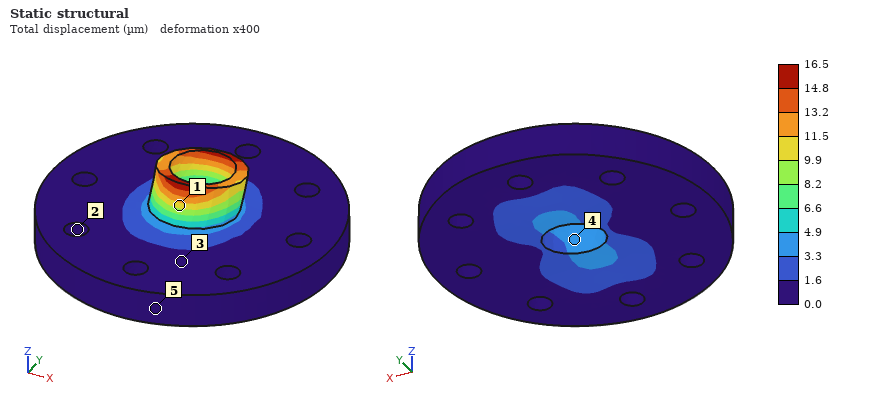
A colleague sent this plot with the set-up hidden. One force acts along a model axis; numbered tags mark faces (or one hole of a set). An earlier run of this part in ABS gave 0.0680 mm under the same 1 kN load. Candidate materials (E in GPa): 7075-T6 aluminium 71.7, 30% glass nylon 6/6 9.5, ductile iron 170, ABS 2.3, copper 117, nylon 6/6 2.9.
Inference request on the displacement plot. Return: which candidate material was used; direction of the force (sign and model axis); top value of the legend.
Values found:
30% glass nylon 6/6
+Y
16.5 µm
